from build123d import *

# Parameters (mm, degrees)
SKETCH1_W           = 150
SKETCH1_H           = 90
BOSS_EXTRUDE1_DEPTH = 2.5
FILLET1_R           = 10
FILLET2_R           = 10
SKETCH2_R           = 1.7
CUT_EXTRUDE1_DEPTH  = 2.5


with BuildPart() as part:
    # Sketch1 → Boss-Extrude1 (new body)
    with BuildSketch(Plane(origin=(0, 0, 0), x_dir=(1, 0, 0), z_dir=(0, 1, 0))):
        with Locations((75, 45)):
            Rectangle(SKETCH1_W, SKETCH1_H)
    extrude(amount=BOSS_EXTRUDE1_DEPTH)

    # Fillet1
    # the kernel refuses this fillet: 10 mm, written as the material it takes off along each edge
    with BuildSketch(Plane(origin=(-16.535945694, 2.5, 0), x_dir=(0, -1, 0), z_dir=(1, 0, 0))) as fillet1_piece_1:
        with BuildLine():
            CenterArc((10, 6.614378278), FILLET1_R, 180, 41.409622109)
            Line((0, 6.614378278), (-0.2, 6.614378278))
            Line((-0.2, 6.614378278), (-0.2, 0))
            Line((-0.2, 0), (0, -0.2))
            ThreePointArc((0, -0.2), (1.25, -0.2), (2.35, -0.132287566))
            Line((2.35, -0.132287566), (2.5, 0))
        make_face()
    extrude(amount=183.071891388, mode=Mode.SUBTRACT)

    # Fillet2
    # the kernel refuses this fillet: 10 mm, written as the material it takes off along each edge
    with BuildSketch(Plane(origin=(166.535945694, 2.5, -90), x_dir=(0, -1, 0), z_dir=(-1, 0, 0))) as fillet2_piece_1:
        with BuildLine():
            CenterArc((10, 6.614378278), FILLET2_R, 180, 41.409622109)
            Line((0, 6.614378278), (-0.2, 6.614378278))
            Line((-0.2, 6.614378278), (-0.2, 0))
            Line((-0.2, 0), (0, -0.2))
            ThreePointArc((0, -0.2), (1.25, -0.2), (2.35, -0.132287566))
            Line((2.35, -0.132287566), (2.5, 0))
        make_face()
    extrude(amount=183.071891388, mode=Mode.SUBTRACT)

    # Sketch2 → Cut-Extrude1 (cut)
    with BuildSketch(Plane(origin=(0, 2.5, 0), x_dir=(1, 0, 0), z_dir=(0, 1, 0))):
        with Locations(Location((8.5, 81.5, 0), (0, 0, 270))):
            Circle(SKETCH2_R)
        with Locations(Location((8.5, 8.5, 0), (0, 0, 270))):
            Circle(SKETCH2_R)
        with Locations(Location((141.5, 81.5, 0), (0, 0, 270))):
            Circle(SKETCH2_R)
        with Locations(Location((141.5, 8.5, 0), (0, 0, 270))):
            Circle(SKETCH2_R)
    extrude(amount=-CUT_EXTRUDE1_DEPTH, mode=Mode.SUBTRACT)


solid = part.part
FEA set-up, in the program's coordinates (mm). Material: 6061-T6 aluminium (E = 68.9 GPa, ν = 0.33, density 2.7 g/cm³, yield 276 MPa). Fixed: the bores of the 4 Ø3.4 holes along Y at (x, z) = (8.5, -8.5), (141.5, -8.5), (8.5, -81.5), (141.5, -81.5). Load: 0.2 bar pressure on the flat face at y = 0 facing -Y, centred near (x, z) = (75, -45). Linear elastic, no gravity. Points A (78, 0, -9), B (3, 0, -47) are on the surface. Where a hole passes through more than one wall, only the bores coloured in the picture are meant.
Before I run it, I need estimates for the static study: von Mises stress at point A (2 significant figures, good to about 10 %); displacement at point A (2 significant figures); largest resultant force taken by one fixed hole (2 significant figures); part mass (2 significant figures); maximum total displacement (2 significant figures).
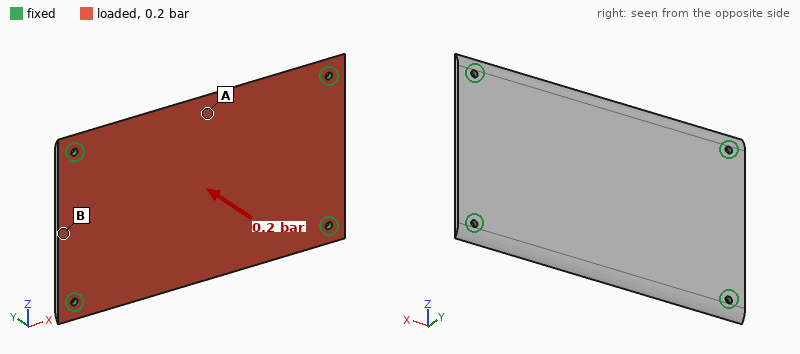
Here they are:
18 MPa
0.27 mm
68 N
87 g
0.28 mm
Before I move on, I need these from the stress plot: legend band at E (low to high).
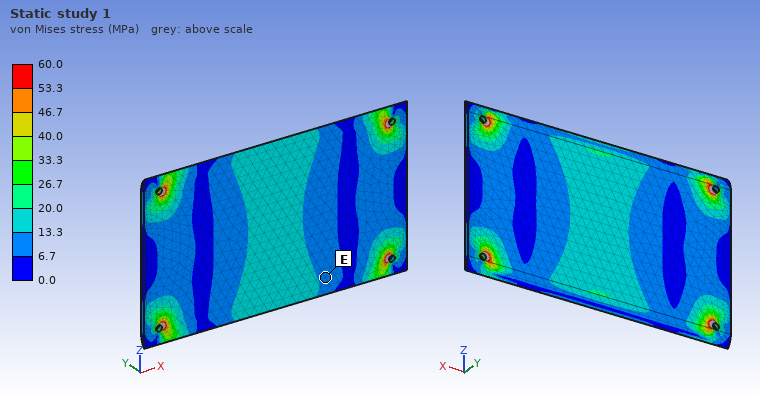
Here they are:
6.7 to 13.3 MPa
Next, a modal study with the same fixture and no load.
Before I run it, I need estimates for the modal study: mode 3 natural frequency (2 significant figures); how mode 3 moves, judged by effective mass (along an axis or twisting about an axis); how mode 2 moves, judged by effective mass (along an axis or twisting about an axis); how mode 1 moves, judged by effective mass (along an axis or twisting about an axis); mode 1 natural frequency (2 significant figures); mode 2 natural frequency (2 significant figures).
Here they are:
1600 Hz
twisting about Z
twisting about X
along Y
610 Hz
1000 Hz
